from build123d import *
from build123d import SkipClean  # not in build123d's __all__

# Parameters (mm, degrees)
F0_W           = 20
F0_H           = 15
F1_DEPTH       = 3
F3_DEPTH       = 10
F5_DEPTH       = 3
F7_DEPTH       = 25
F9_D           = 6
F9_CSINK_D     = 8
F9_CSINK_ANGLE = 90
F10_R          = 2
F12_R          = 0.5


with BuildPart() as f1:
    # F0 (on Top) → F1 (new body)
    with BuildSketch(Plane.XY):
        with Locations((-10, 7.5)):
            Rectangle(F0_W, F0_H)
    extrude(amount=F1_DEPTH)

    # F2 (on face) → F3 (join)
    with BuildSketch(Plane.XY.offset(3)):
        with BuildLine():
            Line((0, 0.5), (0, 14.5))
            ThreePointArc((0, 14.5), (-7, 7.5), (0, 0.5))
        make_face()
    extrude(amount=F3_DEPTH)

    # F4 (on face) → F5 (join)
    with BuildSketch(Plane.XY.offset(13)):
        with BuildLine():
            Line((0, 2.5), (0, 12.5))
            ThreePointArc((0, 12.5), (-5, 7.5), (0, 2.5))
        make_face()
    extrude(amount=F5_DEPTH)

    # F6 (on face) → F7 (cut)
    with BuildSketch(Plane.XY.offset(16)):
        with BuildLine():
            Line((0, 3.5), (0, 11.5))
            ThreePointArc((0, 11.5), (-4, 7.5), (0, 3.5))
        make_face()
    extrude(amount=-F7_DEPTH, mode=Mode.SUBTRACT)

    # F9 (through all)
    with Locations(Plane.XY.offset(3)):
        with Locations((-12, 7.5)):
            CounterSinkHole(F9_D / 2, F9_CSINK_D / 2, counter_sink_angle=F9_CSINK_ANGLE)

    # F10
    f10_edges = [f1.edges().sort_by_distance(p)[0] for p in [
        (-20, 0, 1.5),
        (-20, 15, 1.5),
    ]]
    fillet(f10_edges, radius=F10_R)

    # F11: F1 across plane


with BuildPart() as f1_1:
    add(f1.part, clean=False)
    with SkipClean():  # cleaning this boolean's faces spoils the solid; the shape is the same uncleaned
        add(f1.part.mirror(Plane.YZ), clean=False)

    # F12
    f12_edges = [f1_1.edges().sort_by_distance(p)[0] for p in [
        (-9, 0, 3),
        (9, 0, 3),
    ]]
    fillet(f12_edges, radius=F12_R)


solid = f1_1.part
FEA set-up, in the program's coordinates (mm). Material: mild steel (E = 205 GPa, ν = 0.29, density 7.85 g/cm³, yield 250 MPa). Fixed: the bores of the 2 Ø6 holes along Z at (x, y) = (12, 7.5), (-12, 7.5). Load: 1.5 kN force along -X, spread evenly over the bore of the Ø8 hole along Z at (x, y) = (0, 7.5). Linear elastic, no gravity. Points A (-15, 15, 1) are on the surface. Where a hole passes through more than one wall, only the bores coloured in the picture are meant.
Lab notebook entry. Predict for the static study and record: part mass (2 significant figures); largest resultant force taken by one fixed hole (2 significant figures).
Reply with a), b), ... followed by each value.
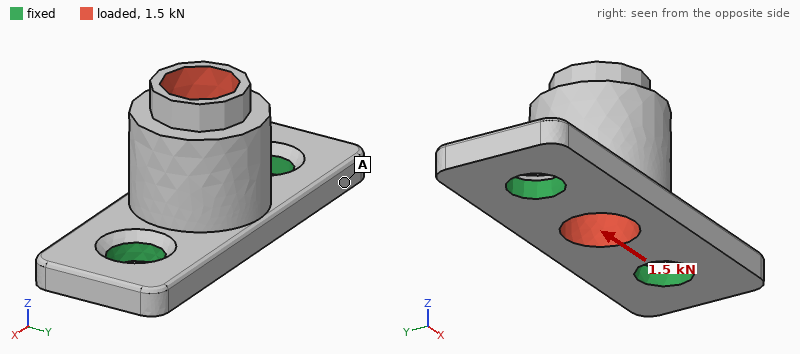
a) 20 g
b) 950 N
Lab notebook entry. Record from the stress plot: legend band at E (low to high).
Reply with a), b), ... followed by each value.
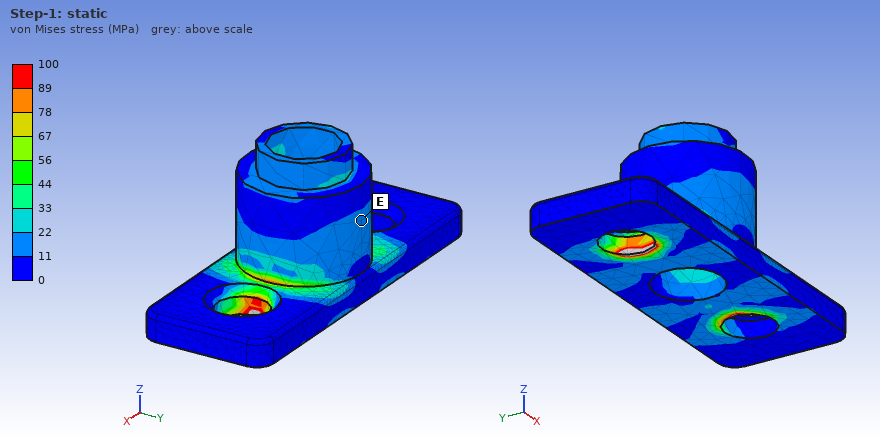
a) 11 to 22 MPa
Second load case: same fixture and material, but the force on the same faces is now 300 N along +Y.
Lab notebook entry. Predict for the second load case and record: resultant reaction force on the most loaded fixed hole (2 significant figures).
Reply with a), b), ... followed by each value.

a) 150 N
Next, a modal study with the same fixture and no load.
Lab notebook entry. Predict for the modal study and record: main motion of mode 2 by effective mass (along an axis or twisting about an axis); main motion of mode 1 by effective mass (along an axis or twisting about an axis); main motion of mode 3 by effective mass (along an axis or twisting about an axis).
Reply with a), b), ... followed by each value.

a) along Z
b) along Y
c) along X
